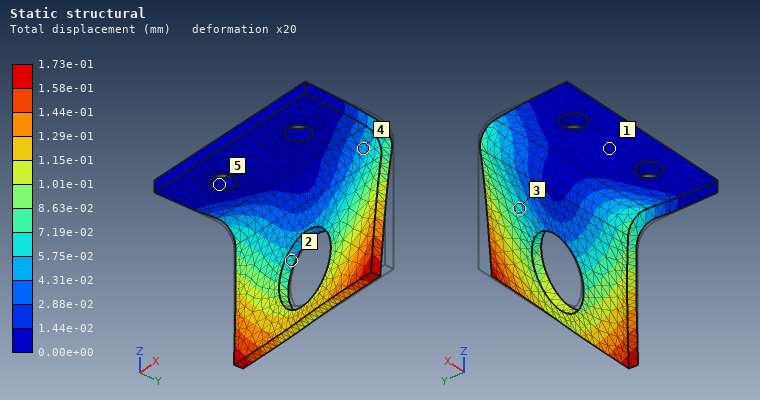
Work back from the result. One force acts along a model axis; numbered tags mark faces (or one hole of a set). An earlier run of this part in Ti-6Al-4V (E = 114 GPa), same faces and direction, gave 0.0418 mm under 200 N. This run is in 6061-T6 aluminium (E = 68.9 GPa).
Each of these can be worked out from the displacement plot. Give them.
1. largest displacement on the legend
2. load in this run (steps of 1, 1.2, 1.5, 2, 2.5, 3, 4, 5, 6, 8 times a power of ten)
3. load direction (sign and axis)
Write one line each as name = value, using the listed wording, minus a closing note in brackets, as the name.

largest displacement on the legend = 1.73e-01 mm
load in this run = 500 N
load direction = -X
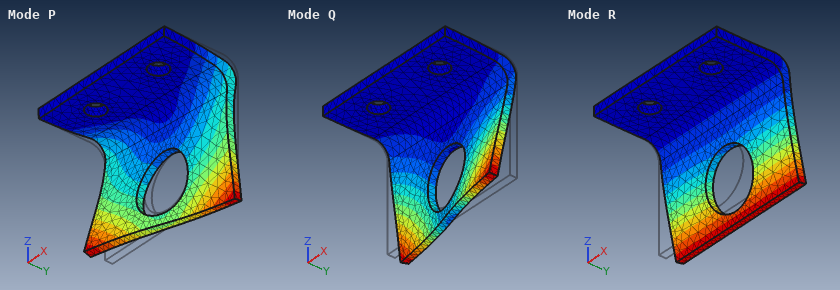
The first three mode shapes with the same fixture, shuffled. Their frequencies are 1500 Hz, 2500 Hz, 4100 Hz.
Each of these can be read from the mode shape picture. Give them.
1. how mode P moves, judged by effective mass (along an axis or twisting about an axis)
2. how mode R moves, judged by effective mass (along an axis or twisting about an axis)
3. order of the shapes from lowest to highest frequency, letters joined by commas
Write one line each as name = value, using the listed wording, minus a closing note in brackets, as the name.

how mode P moves, judged by effective mass = along X
how mode R moves, judged by effective mass = along Y
order of the shapes from lowest to highest frequency, letters joined by commas = R, Q, P
